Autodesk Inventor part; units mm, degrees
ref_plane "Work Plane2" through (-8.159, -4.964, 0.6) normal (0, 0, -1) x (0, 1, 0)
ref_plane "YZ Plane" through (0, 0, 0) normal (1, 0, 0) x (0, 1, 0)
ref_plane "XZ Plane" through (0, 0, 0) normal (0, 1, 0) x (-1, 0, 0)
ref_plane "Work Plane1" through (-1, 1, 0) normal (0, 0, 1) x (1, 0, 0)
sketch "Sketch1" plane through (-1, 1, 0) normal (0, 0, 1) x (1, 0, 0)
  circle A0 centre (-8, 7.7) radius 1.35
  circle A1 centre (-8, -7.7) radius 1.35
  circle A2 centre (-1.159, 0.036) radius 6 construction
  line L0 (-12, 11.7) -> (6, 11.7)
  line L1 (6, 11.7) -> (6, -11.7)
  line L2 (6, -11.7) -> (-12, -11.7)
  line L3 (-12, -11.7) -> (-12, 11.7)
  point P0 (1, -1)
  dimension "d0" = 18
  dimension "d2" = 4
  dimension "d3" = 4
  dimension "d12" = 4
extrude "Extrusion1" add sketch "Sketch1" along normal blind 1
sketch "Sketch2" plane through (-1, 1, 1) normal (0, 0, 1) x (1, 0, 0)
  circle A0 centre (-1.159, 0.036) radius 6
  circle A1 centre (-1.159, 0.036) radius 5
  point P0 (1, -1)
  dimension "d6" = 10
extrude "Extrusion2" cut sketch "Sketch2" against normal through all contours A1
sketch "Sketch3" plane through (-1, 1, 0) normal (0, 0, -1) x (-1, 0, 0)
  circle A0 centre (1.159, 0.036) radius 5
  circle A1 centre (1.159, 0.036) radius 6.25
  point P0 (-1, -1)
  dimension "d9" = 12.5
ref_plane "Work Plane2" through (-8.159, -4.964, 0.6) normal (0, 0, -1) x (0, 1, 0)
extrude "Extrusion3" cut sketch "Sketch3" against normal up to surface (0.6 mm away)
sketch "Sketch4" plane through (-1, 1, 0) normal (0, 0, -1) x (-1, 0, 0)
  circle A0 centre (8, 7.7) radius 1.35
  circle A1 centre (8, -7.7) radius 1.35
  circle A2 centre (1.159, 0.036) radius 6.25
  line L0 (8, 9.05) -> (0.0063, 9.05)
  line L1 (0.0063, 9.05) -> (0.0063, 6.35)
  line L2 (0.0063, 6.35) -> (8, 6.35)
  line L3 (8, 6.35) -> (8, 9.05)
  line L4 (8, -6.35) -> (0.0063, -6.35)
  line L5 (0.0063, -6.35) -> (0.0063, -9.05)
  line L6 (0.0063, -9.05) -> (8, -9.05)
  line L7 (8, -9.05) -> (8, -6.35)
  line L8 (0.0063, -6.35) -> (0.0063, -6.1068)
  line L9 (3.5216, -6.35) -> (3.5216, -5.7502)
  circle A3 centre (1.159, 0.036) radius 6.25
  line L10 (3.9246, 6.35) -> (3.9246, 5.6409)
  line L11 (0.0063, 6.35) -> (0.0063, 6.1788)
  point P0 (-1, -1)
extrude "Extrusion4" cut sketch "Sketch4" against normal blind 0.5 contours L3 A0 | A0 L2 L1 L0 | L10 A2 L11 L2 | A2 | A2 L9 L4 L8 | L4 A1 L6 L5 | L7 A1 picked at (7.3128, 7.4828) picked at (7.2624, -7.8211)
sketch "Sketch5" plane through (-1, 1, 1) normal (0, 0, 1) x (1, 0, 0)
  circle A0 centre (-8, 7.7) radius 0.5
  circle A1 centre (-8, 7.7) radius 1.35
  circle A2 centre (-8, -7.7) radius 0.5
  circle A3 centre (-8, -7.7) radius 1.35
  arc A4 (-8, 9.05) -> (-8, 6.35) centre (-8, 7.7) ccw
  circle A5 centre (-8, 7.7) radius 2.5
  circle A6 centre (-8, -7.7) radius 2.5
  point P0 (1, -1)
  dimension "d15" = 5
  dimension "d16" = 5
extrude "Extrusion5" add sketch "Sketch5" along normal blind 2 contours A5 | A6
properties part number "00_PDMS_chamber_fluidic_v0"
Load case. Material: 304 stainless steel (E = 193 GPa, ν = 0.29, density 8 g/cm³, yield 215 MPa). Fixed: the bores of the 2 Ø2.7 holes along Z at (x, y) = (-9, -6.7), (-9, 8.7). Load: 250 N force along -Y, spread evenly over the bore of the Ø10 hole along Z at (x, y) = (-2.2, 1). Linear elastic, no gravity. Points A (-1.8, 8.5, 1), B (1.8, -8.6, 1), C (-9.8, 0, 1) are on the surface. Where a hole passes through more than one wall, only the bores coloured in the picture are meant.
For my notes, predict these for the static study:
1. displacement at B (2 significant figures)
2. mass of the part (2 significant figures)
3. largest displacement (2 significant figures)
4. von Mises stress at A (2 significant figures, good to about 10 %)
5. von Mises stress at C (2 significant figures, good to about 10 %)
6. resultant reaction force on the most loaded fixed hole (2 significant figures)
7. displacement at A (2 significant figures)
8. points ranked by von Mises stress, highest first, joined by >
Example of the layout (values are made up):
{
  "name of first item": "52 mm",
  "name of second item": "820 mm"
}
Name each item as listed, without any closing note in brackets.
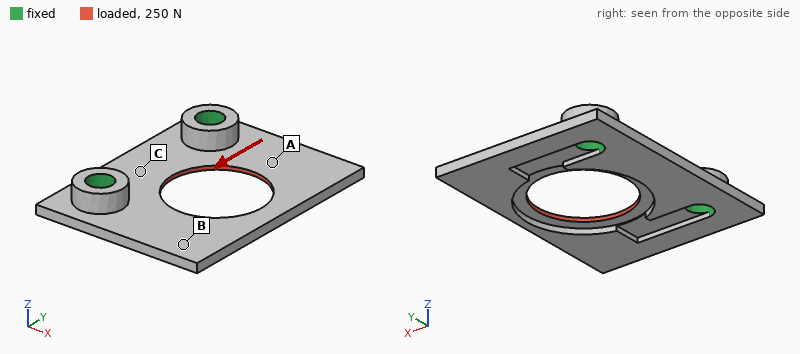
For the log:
{
  "displacement at B": "6.9 µm",
  "mass of the part": "2.7 g",
  "largest displacement": "9.9 µm",
  "von Mises stress at A": "48 MPa",
  "von Mises stress at C": "18 MPa",
  "resultant reaction force on the most loaded fixed hole": "140 N",
  "displacement at A": "3.9 µm",
  "points ranked by von Mises stress, highest first, joined by >": "A > C > B"
}
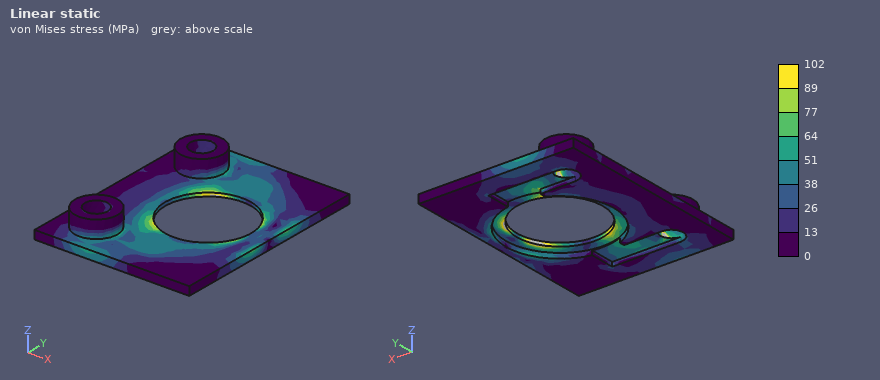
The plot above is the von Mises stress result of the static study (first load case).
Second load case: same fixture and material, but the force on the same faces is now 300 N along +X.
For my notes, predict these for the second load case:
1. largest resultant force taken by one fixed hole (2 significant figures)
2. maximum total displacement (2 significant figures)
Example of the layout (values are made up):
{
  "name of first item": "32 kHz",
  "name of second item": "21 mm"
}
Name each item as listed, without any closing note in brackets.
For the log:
{
  "largest resultant force taken by one fixed hole": "150 N",
  "maximum total displacement": "13 µm"
}
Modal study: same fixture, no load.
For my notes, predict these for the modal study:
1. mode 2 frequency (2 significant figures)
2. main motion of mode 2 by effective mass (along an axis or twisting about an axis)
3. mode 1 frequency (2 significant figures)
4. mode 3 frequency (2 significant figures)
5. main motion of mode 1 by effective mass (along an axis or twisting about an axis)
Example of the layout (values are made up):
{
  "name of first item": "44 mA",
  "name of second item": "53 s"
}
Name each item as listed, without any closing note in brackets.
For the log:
{
  "mode 2 frequency": "5300 Hz",
  "main motion of mode 2 by effective mass": "twisting about X",
  "mode 1 frequency": "3300 Hz",
  "mode 3 frequency": "11 kHz",
  "main motion of mode 1 by effective mass": "along Z"
}
